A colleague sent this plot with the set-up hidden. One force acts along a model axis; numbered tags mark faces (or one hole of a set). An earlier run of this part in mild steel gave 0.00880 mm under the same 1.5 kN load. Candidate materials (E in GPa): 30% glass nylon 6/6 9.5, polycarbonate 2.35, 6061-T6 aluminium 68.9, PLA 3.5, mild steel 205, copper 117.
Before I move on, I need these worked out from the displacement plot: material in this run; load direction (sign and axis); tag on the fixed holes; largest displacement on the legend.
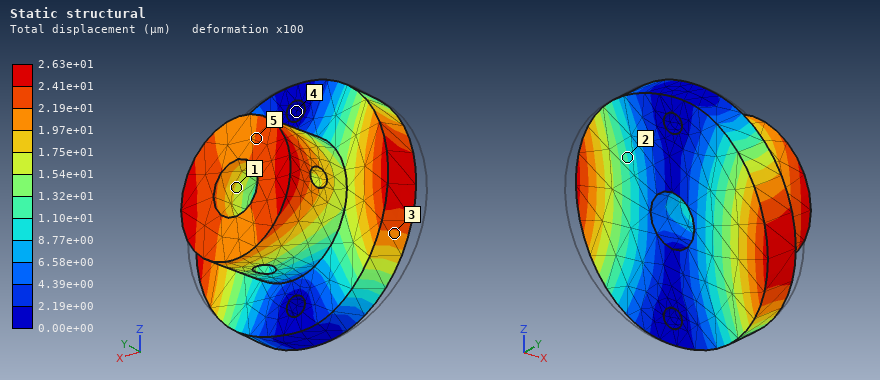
6061-T6 aluminium
+X
4
2.63e+01 µm
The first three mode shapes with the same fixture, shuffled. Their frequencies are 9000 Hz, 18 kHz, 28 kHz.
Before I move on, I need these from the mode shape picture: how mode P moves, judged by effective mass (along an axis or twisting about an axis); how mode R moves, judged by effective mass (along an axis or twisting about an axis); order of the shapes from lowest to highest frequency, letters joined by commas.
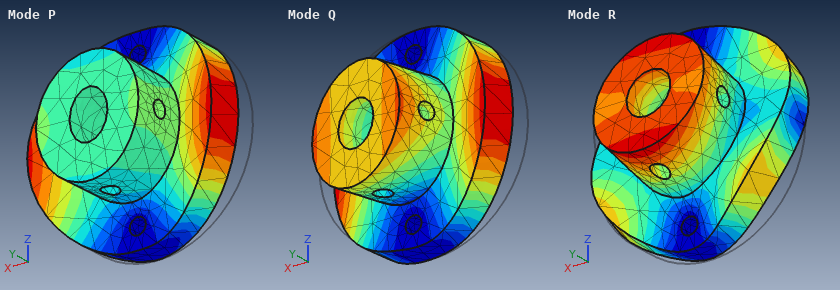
along Y
along Z
Q, P, R
